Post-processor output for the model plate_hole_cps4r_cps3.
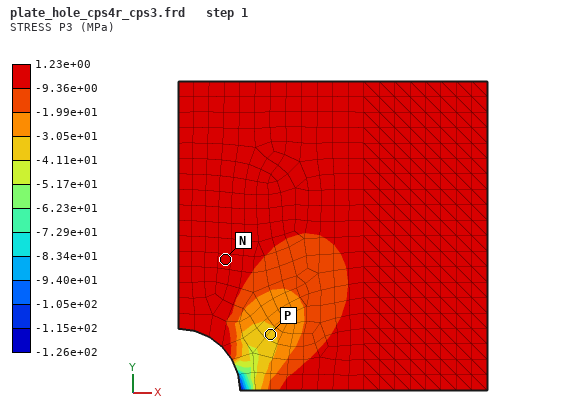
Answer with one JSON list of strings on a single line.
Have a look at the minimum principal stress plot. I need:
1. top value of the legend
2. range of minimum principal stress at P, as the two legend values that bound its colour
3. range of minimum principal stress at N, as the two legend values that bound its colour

["1.23e+00 MPa", "-4.11e+01 to -3.05e+01 MPa", "-9.36e+00 to 1.23e+00 MPa"]
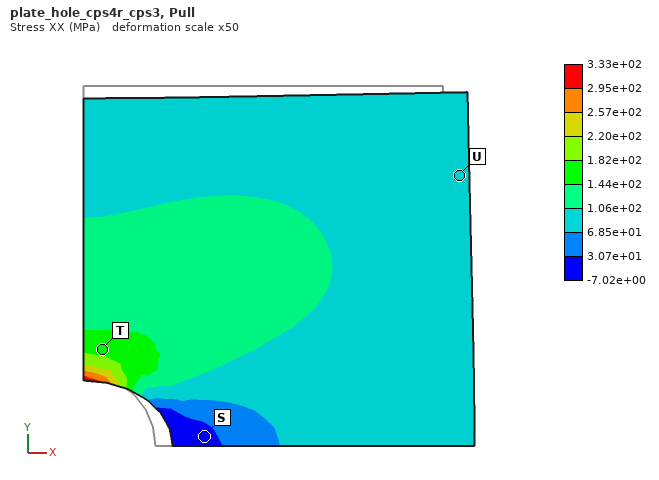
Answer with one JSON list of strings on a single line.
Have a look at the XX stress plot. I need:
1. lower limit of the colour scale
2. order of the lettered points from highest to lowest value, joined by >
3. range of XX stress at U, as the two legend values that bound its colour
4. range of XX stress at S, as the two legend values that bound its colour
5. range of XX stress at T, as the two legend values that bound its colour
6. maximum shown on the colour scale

["-7.02e+00 MPa", "T > U > S", "6.85e+01 to 1.06e+02 MPa", "-7.02e+00 to 3.07e+01 MPa", "1.44e+02 to 1.82e+02 MPa", "3.33e+02 MPa"]
